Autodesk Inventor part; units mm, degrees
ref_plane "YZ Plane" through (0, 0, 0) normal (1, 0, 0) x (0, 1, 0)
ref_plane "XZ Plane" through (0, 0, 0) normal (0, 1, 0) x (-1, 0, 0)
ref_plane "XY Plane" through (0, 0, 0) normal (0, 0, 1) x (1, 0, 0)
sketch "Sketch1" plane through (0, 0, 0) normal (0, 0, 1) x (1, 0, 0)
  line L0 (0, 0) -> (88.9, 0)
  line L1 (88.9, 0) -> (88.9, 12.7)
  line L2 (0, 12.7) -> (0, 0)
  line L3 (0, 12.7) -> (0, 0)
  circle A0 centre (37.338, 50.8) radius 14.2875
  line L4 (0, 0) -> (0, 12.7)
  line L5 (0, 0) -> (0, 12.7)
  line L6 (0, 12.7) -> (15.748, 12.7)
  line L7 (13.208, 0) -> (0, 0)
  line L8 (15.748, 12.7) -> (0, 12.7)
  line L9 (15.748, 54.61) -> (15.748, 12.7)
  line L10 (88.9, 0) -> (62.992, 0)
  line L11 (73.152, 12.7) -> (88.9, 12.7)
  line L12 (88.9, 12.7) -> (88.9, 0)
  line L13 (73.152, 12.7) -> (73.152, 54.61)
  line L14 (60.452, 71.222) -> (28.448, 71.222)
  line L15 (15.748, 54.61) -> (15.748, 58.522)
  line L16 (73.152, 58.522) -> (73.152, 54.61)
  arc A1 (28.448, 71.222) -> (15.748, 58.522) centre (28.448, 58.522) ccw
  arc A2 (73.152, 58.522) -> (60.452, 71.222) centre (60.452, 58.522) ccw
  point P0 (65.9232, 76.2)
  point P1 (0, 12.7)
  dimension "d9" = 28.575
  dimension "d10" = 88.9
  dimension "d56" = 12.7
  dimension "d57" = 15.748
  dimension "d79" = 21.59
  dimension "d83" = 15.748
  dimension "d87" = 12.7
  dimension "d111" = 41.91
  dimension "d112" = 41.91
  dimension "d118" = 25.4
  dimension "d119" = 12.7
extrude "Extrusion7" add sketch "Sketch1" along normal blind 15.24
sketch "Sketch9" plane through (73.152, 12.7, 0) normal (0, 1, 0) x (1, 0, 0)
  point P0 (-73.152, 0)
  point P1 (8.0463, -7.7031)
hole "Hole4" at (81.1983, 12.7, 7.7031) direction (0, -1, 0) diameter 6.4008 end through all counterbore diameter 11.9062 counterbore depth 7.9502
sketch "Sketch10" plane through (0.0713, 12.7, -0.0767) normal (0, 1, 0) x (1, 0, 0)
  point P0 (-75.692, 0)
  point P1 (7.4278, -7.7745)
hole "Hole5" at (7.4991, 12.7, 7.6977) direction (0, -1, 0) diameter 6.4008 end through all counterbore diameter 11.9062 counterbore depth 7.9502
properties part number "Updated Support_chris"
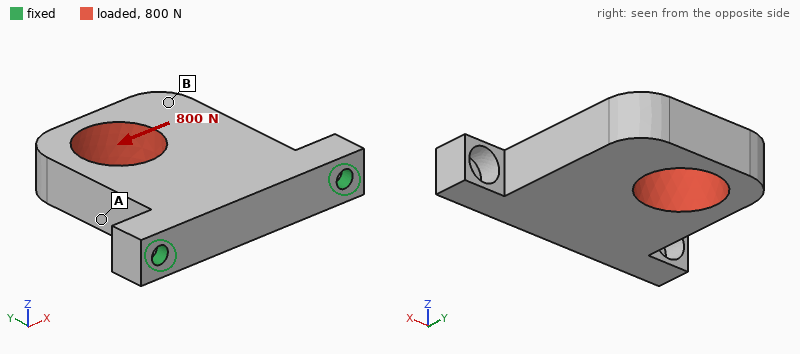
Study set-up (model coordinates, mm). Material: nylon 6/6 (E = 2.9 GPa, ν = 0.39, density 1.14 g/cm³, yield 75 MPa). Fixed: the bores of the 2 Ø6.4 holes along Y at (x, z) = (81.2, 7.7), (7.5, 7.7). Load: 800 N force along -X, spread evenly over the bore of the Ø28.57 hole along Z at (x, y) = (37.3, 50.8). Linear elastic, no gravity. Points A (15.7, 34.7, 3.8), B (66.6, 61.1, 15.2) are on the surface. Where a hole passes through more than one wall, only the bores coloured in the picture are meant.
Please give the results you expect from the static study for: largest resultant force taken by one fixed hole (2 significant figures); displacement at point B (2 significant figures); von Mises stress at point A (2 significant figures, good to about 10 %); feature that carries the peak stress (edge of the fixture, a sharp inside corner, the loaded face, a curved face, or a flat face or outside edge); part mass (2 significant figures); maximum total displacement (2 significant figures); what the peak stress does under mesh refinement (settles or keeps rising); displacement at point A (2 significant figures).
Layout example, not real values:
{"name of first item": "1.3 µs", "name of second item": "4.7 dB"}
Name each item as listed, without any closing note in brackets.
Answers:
{"largest resultant force taken by one fixed hole": "700 N", "displacement at point B": "0.27 mm", "von Mises stress at point A": "4.4 MPa", "feature that carries the peak stress": "edge of the fixture", "part mass": "63 g", "maximum total displacement": "0.32 mm", "what the peak stress does under mesh refinement": "keeps rising", "displacement at point A": "0.15 mm"}
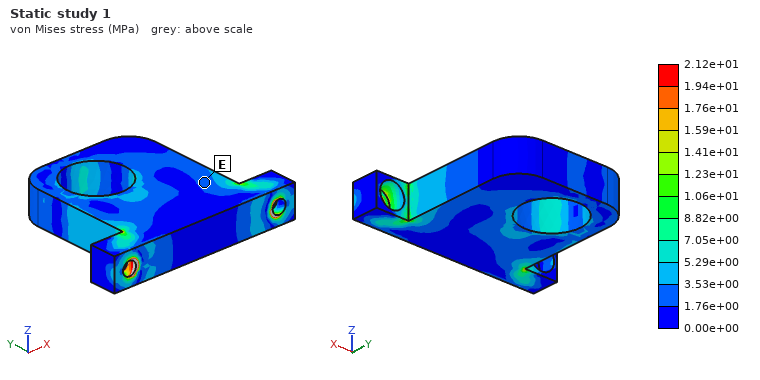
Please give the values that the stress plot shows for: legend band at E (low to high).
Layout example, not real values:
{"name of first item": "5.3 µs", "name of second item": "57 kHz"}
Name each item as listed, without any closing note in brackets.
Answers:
{"legend band at E": "1.76e+00 to 3.53e+00 MPa"}
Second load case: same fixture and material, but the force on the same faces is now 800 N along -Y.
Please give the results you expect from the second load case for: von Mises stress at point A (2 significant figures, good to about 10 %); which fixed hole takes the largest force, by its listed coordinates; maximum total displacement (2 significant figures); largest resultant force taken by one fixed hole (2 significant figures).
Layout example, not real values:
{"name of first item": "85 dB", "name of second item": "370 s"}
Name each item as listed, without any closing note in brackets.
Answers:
{"von Mises stress at point A": "3.1 MPa", "which fixed hole takes the largest force, by its listed coordinates": "(7.5, 7.7)", "maximum total displacement": "0.13 mm", "largest resultant force taken by one fixed hole": "550 N"}
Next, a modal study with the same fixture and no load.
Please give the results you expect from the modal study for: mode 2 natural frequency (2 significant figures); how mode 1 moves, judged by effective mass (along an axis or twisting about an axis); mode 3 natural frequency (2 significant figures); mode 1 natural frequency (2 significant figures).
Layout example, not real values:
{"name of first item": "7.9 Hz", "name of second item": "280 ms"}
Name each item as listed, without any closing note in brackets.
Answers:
{"mode 2 natural frequency": "1600 Hz", "how mode 1 moves, judged by effective mass": "along Z", "mode 3 natural frequency": "1700 Hz", "mode 1 natural frequency": "350 Hz"}
